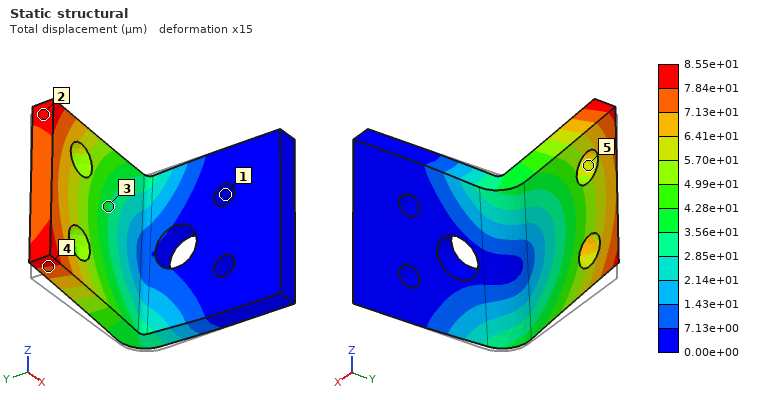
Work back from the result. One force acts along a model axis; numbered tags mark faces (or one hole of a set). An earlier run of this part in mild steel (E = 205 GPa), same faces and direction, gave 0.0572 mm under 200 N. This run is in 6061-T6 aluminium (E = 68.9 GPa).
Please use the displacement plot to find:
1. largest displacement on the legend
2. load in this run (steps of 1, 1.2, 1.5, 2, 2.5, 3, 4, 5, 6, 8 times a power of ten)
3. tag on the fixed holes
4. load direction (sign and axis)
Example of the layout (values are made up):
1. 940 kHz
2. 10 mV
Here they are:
1. 8.55e+01 µm
2. 100 N
3. 1
4. +Z
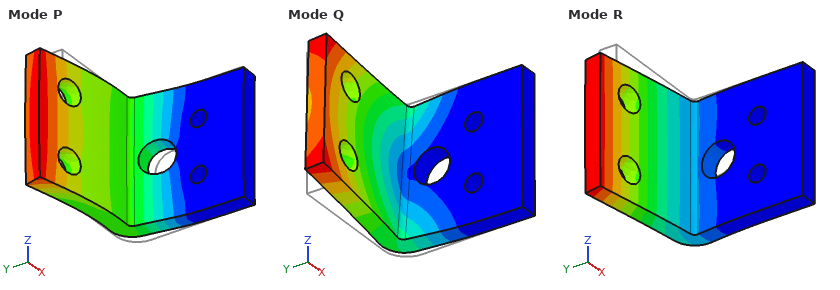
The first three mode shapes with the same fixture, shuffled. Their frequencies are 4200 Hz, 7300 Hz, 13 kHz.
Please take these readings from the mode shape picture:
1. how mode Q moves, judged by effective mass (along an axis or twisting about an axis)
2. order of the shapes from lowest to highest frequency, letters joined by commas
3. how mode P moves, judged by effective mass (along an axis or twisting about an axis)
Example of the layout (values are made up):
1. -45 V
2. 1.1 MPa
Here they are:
1. along Z
2. R, Q, P
3. along X
